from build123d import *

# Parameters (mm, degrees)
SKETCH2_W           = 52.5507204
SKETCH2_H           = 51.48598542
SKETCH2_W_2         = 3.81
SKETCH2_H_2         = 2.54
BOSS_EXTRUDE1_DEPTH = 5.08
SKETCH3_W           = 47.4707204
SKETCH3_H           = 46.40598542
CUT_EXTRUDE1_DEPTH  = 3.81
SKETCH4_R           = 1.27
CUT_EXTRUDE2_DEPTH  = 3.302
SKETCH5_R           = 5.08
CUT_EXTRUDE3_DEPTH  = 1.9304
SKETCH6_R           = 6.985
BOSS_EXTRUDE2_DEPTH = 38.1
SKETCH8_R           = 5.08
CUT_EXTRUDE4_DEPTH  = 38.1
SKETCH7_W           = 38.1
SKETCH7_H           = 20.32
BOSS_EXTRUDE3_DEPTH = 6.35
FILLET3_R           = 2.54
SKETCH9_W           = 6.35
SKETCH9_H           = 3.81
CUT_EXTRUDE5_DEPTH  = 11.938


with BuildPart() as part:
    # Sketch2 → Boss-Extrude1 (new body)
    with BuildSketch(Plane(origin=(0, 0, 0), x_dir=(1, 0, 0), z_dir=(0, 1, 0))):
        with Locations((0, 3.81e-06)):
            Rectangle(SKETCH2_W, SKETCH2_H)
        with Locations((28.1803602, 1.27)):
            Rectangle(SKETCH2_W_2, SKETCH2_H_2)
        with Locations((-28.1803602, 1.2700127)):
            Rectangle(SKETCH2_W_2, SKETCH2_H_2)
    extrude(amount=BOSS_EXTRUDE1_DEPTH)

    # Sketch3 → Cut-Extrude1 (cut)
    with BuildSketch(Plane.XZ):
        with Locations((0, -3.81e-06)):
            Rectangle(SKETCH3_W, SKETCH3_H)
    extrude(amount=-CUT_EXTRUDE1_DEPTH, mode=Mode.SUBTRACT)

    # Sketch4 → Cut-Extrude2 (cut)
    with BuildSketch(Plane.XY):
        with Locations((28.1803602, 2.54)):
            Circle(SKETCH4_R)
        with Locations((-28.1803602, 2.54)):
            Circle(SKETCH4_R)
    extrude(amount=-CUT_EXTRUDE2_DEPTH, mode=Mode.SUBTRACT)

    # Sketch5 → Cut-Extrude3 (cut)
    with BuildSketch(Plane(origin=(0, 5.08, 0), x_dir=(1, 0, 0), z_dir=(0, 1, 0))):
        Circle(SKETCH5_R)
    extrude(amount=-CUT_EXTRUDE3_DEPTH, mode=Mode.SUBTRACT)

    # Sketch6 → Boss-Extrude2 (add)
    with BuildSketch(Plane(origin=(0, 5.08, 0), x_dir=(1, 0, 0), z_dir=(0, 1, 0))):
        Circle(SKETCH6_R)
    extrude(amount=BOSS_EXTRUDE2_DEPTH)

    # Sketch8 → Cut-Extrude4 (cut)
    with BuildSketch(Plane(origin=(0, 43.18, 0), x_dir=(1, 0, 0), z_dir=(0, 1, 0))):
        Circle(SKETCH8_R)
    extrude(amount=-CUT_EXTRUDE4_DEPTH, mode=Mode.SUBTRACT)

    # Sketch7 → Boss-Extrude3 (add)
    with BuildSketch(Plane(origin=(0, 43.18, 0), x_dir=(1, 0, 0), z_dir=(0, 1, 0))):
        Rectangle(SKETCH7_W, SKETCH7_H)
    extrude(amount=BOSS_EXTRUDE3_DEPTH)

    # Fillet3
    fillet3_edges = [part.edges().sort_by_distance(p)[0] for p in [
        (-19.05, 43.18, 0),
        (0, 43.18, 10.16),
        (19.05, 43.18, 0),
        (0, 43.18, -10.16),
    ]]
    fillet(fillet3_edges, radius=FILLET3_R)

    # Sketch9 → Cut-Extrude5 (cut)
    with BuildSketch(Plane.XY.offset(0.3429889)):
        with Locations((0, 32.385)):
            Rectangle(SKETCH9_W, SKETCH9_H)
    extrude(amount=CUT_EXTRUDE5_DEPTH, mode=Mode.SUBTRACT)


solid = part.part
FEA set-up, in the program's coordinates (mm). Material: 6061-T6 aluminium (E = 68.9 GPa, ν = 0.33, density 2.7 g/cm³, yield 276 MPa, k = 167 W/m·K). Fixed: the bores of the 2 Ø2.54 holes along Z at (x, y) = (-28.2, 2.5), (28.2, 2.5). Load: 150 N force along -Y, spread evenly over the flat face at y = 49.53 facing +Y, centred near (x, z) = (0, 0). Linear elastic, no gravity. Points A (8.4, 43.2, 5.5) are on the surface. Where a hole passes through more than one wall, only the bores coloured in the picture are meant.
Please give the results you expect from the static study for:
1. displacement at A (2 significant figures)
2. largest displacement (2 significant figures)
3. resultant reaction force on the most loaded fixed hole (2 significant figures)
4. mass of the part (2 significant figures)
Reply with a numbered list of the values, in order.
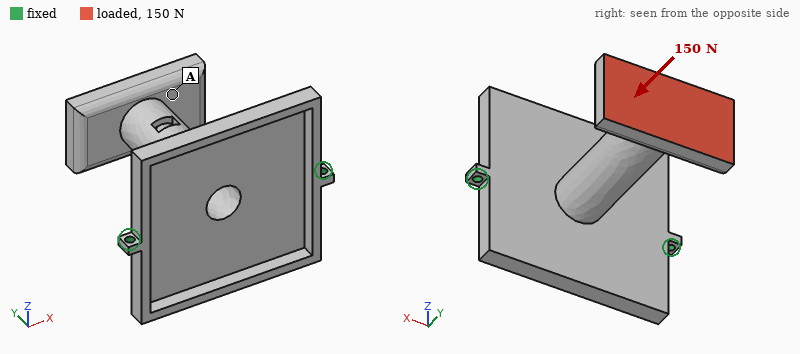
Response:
1. 0.11 mm
2. 0.11 mm
3. 130 N
4. 35 g
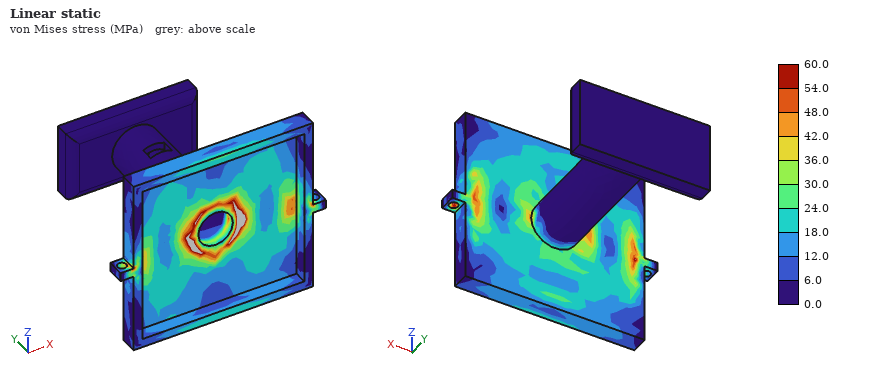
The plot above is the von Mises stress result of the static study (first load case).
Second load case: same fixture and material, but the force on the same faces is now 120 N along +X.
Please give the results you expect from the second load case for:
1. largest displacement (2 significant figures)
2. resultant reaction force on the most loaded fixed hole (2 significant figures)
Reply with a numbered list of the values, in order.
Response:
1. 0.96 mm
2. 150 N
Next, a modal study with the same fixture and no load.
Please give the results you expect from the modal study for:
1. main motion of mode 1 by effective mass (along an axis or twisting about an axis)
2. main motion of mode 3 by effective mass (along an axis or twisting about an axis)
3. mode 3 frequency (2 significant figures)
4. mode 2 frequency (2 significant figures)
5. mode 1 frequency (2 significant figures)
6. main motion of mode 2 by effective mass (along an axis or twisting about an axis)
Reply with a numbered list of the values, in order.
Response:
1. along Z
2. along Y
3. 1300 Hz
4. 500 Hz
5. 380 Hz
6. along X
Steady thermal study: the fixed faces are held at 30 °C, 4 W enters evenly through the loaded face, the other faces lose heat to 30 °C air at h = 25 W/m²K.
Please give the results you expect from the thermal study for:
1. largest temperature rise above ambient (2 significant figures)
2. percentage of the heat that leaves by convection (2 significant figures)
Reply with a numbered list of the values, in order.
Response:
1. 16 K
2. 45 %
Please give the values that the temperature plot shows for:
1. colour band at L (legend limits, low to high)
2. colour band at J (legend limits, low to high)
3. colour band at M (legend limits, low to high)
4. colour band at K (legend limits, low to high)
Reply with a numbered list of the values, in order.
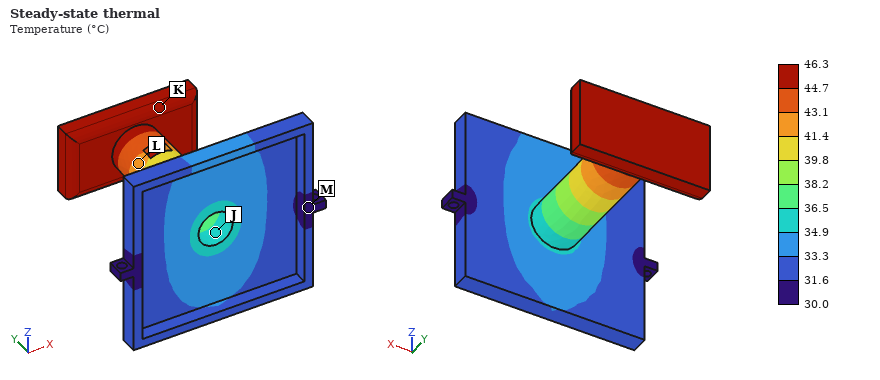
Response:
1. 41.4 to 43.1 °C
2. 34.9 to 36.5 °C
3. 30.0 to 31.6 °C
4. 44.7 to 46.3 °C
